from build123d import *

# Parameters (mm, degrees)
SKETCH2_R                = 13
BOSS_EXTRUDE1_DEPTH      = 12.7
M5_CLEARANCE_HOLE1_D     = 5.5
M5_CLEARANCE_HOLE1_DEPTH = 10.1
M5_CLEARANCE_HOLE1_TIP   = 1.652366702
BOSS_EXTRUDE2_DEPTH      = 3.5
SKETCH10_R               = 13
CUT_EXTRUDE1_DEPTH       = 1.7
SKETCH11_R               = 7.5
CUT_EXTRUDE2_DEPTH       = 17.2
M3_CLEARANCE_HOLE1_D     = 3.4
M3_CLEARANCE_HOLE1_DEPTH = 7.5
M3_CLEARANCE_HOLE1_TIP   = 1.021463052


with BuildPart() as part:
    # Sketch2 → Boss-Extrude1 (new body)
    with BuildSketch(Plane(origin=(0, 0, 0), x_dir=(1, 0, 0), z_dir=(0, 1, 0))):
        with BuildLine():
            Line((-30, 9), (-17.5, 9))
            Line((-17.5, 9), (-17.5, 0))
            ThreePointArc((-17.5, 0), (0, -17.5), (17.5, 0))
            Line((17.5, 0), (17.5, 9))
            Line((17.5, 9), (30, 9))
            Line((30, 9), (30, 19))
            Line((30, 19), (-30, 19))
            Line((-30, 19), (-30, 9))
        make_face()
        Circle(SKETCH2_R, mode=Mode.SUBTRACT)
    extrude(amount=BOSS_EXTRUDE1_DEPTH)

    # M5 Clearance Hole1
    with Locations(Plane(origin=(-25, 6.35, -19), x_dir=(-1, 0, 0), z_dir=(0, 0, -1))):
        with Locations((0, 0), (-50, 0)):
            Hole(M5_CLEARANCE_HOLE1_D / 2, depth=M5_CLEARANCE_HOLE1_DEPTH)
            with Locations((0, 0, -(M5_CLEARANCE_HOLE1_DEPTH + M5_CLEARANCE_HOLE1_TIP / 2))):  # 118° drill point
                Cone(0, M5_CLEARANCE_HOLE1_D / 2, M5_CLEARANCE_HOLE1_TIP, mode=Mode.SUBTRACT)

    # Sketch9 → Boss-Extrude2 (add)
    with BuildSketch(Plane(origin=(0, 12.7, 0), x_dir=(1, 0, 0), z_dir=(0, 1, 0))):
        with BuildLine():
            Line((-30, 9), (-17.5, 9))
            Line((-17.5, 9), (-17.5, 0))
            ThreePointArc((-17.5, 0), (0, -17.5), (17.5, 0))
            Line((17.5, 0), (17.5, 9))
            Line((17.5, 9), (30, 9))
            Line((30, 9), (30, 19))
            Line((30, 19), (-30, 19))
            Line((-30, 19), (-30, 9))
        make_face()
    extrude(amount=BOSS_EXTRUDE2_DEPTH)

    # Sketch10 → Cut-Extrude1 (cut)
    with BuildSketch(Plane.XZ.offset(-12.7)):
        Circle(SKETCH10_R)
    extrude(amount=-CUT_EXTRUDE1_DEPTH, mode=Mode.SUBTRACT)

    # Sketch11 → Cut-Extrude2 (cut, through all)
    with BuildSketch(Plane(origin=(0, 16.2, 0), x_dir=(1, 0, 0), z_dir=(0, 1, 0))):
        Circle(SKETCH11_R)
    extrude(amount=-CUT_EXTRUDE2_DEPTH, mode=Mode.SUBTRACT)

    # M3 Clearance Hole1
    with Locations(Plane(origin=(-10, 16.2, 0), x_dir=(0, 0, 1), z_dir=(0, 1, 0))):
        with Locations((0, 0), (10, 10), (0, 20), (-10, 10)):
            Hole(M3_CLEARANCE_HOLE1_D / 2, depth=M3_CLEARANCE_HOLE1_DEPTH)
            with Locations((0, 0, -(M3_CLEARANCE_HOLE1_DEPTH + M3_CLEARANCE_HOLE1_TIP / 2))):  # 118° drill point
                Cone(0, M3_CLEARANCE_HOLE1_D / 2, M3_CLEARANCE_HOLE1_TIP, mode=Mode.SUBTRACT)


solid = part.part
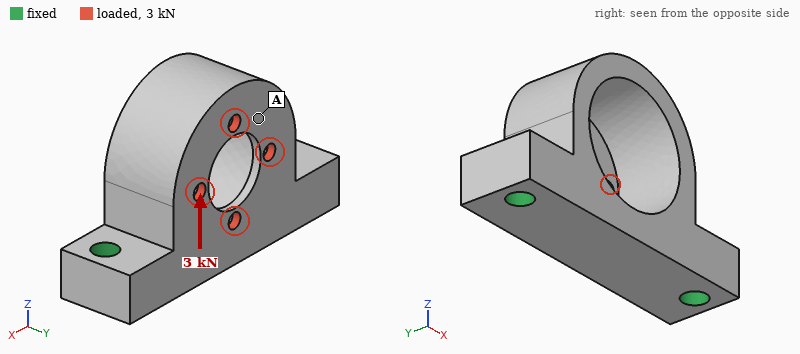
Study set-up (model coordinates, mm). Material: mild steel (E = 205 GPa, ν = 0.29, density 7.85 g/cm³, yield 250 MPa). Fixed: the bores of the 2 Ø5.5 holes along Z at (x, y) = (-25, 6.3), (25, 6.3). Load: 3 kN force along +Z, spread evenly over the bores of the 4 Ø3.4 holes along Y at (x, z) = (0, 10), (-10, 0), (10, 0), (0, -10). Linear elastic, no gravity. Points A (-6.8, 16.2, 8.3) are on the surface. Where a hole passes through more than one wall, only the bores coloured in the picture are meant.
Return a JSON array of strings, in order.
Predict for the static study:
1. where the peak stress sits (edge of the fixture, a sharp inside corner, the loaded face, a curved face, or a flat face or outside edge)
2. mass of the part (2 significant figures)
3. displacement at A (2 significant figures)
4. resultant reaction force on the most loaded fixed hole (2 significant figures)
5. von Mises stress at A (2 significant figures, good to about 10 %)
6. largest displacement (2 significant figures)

["a curved face", "110 g", "16 µm", "1.5 kN", "18 MPa", "23 µm"]
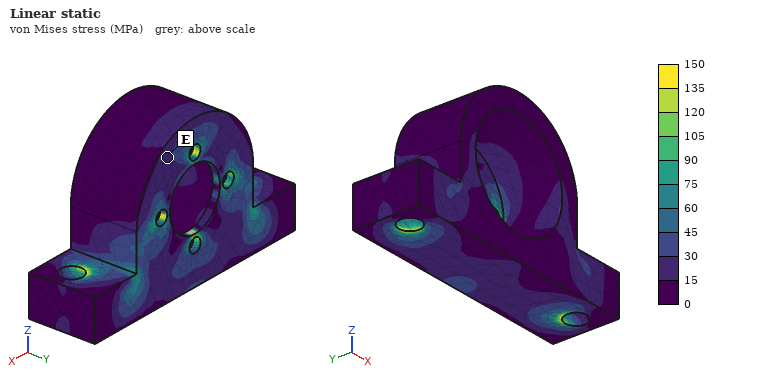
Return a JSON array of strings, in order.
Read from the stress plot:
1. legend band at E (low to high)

["15 to 30 MPa"]
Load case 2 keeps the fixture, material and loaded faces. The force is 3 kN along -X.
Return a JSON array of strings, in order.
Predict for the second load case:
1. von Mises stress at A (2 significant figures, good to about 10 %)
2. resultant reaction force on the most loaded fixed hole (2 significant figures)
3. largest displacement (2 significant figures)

["27 MPa", "1.8 kN", "15 µm"]
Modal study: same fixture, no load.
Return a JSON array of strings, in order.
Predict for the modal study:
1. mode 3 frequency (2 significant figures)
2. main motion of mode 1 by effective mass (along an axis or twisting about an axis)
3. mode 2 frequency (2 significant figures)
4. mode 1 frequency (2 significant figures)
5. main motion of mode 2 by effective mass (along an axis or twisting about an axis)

["16 kHz", "along Y", "9900 Hz", "6800 Hz", "along X"]
